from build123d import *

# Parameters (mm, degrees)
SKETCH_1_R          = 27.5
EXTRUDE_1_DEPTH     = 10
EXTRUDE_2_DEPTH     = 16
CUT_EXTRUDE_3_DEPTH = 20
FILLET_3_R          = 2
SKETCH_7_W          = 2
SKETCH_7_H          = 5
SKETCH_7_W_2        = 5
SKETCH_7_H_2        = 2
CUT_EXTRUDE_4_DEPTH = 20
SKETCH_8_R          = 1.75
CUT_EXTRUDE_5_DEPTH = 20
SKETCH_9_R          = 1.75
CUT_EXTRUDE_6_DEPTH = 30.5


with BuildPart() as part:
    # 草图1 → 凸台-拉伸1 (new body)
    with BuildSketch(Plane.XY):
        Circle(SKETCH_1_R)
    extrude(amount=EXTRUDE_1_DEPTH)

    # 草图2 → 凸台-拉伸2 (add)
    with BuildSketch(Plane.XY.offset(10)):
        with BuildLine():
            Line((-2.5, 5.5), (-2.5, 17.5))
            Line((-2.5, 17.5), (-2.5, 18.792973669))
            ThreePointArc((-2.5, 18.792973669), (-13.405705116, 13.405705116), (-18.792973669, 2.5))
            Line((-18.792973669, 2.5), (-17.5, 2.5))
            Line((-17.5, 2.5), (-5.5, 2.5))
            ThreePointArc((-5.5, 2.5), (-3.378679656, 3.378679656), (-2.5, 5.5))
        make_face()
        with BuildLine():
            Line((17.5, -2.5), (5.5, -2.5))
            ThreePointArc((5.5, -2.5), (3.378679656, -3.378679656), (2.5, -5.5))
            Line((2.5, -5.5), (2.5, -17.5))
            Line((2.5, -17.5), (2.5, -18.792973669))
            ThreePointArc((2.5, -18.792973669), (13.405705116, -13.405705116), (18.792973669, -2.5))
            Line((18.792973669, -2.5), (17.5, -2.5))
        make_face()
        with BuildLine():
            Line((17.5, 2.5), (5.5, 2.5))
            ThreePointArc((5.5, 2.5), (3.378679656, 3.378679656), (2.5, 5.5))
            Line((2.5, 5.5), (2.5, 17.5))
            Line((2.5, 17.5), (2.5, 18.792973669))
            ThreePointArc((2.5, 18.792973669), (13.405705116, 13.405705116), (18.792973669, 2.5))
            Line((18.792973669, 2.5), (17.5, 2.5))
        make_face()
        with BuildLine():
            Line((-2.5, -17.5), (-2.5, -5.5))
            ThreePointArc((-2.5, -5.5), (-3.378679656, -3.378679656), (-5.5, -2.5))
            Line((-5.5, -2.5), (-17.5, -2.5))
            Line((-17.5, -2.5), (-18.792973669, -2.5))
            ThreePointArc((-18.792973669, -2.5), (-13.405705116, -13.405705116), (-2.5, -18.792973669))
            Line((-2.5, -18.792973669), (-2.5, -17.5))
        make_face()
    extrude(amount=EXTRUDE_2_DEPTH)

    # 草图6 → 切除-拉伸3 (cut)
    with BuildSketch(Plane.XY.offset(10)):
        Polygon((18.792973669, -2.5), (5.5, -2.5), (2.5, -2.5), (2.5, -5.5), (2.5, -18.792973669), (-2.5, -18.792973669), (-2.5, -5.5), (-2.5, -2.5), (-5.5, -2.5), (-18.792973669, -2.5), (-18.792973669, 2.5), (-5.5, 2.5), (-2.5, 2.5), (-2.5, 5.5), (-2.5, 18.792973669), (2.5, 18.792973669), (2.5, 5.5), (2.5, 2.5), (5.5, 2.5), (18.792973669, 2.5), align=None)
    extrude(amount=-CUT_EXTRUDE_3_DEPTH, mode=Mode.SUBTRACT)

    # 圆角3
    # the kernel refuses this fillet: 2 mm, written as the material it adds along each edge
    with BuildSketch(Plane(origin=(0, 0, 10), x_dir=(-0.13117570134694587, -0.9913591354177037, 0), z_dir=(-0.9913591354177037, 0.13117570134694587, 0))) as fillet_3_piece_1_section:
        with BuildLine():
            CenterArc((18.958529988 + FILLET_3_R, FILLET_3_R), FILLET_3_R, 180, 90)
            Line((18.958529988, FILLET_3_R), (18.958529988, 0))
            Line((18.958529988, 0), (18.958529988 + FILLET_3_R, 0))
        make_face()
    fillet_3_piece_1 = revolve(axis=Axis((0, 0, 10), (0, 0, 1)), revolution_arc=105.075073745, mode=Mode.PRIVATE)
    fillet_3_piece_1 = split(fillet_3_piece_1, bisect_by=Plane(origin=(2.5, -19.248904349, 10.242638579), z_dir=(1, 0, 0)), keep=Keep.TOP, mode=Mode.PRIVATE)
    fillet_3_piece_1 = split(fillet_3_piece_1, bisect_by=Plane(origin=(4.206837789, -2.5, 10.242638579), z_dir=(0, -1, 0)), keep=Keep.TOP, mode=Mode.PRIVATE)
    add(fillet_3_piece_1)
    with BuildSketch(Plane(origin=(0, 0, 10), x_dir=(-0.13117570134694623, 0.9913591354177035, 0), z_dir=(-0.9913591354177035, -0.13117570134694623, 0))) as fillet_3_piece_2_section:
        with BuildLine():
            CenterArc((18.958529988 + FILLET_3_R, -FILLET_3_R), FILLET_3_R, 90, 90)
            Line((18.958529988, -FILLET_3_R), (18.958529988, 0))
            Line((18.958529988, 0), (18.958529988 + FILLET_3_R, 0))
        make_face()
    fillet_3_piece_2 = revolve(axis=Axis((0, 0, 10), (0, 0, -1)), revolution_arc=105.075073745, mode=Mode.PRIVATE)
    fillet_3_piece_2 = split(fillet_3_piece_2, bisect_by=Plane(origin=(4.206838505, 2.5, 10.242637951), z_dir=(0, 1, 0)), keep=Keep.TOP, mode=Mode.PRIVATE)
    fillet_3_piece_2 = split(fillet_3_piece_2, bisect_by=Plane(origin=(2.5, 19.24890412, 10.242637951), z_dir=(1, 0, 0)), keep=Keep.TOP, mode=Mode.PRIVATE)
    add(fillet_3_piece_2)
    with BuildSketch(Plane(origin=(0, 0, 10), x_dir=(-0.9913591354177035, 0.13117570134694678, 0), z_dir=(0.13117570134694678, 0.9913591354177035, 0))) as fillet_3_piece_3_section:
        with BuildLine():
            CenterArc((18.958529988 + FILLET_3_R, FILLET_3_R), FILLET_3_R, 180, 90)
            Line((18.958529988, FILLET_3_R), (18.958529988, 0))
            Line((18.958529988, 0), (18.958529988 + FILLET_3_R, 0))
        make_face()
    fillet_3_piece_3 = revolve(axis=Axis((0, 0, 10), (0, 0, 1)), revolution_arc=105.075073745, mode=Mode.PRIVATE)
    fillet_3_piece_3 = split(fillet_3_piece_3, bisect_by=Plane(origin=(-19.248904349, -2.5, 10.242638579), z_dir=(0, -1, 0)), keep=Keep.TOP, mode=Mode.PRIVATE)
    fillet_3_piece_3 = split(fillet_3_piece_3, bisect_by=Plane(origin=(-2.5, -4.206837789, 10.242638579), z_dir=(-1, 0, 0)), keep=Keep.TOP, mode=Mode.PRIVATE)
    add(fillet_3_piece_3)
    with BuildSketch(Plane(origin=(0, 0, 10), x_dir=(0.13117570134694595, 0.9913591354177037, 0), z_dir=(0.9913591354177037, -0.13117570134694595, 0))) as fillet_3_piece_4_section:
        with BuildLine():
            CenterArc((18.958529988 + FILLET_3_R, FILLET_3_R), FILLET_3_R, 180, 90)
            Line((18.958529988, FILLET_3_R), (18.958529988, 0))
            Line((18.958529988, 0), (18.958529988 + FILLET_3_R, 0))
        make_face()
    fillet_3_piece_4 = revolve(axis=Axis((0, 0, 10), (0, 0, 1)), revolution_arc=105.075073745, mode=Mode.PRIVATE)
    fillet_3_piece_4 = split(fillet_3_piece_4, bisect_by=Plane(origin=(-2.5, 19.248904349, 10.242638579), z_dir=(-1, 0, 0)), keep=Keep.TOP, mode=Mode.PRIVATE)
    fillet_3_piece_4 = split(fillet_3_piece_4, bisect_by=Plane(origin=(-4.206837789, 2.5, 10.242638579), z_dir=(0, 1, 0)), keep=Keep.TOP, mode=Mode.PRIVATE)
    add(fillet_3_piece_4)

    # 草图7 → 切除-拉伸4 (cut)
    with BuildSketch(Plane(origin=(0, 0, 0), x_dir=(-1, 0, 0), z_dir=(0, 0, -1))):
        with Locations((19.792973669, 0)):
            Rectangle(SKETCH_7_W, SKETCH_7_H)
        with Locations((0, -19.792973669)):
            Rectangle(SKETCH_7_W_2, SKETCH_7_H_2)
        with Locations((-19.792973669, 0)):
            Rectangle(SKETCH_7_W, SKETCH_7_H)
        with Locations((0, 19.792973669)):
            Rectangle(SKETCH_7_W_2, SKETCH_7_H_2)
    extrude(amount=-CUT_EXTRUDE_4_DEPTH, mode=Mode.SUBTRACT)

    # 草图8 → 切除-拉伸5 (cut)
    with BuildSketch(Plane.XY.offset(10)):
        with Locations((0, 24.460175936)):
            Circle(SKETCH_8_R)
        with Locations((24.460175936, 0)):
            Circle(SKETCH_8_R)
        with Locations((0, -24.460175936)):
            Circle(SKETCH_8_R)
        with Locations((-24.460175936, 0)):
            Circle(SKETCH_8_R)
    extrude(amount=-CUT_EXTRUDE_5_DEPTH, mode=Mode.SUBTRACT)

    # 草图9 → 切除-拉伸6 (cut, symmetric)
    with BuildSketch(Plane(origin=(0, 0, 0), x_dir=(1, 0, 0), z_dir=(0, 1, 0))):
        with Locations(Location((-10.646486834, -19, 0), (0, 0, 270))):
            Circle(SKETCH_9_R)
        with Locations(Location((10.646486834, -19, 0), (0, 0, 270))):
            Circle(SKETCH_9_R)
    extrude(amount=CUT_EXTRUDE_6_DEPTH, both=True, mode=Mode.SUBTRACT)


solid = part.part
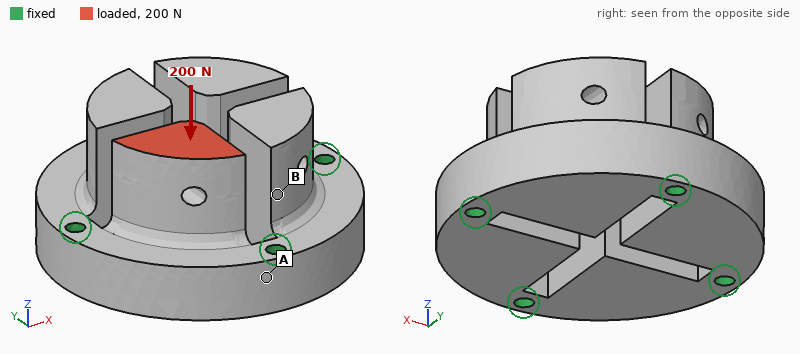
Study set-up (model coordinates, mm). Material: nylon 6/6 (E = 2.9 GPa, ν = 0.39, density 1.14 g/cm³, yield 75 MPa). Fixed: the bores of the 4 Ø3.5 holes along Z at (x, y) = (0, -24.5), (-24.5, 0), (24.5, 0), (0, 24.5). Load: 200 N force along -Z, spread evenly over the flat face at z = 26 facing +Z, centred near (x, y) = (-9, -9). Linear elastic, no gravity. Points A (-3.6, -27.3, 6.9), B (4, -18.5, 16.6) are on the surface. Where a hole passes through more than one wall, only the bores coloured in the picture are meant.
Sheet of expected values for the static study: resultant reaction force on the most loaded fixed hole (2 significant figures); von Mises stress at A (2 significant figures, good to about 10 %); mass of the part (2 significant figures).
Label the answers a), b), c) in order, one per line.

a) 100 N
b) 3.0 MPa
c) 36 g
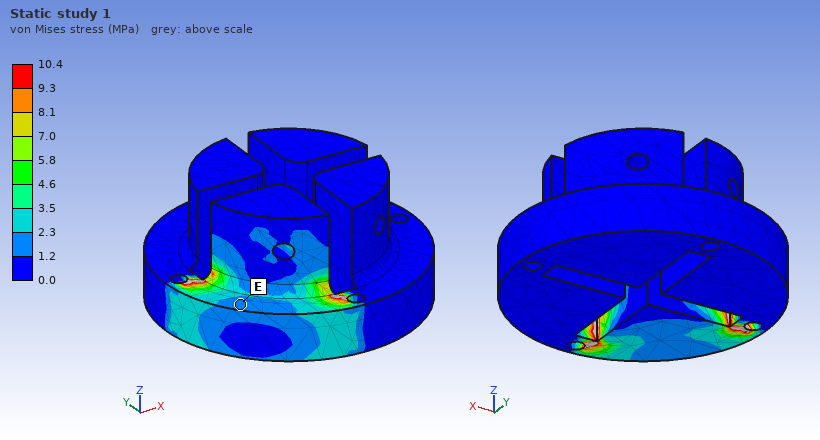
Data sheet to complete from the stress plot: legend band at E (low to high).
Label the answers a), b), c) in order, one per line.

a) 1.2 to 2.3 MPa
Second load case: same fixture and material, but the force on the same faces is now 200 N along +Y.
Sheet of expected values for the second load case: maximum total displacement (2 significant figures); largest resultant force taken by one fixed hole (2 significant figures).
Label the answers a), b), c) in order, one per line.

a) 0.44 mm
b) 150 N
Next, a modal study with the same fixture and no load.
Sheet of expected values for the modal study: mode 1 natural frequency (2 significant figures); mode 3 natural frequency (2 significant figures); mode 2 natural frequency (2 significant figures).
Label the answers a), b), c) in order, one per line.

a) 2200 Hz
b) 2200 Hz
c) 2200 Hz
